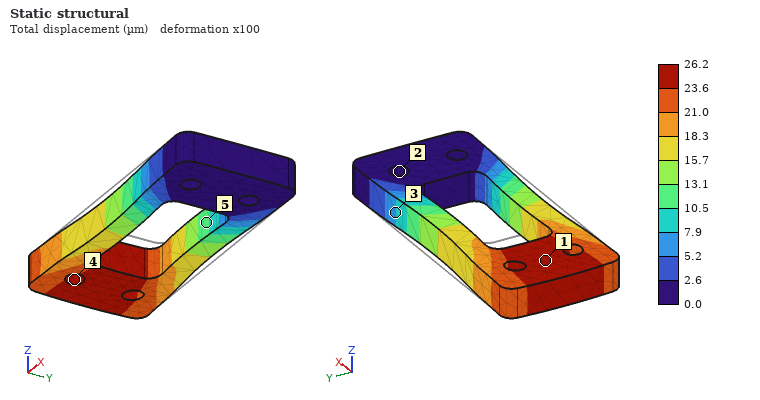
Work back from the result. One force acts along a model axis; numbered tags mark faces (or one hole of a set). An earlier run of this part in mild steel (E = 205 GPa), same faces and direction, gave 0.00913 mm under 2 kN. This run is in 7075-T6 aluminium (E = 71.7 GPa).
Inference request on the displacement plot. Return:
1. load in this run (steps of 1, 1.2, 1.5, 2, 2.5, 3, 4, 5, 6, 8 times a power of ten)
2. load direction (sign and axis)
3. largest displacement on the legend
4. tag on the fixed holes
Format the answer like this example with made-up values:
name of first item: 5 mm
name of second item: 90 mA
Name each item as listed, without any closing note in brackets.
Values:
load in this run: 2 kN
load direction: -X
largest displacement on the legend: 26.2 µm
tag on the fixed holes: 2
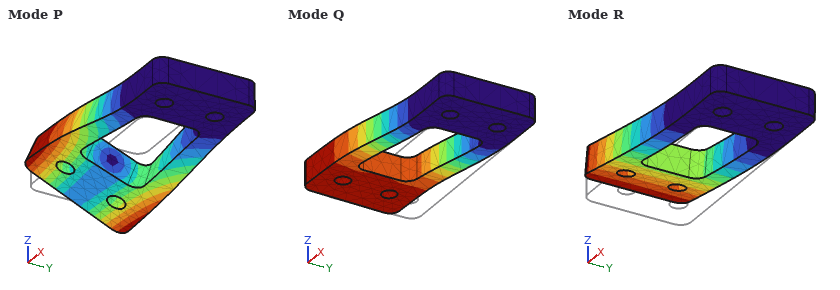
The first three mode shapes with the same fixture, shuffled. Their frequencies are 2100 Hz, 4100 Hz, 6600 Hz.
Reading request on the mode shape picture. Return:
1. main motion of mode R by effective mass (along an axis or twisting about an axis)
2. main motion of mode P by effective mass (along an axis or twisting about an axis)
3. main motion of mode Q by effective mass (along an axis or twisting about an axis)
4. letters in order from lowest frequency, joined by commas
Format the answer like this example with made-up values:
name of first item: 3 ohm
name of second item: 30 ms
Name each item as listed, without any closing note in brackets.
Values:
main motion of mode R by effective mass: along Z
main motion of mode P by effective mass: twisting about X
main motion of mode Q by effective mass: along Y
letters in order from lowest frequency, joined by commas: R, Q, P
